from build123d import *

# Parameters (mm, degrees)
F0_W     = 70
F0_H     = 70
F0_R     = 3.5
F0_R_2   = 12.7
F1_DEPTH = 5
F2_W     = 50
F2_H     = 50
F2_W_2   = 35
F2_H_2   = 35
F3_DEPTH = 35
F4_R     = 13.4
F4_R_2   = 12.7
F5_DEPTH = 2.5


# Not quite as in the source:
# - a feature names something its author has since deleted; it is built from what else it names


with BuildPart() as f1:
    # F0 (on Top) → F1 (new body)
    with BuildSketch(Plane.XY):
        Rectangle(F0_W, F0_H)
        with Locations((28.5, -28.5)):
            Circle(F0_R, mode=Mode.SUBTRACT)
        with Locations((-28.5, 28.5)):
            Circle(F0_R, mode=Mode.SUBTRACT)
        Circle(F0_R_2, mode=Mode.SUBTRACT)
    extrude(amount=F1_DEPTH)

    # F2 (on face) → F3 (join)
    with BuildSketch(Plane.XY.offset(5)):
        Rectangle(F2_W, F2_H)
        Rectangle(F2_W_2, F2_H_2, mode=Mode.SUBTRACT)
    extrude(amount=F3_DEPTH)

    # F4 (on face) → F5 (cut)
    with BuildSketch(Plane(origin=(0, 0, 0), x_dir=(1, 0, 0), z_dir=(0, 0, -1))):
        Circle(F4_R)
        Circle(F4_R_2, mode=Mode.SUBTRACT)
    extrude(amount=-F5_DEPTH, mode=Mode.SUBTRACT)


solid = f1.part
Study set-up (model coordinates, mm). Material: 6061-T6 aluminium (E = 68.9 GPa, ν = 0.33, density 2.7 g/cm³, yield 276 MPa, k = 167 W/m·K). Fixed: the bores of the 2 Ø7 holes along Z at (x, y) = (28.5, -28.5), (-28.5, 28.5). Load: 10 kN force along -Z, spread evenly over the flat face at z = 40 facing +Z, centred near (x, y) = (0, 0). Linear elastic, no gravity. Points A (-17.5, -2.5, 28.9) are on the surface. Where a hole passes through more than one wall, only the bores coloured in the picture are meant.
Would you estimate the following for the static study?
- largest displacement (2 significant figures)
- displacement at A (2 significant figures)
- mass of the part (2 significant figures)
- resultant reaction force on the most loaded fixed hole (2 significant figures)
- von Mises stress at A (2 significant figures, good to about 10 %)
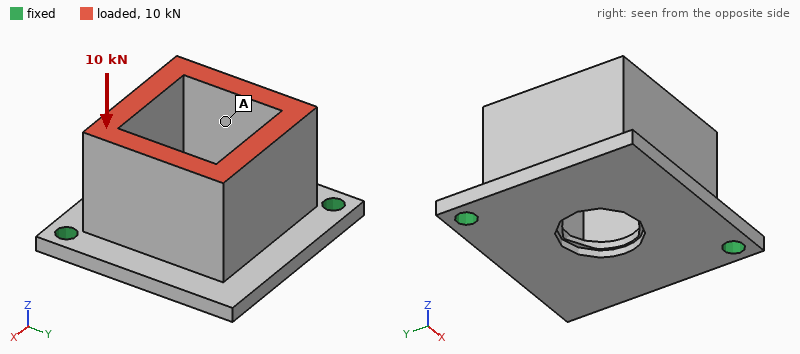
0.15 mm
0.094 mm
180 g
5.6 kN
22 MPa
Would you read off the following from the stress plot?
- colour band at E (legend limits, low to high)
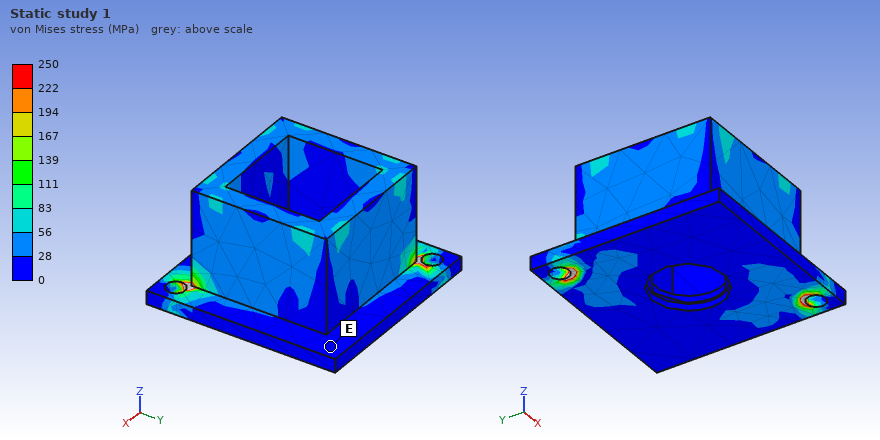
0 to 28 MPa
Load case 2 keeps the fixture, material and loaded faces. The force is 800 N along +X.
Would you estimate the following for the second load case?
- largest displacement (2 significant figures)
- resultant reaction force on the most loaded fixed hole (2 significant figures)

0.17 mm
500 N
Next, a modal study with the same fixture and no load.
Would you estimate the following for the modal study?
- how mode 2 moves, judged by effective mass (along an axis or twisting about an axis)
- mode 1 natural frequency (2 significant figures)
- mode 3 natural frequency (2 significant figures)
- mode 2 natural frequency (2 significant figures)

along Z
1200 Hz
7400 Hz
3800 Hz
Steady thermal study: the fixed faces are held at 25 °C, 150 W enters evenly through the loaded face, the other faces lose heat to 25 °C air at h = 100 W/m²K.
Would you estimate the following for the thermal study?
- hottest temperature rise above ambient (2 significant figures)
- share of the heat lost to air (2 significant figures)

49 K
44 %
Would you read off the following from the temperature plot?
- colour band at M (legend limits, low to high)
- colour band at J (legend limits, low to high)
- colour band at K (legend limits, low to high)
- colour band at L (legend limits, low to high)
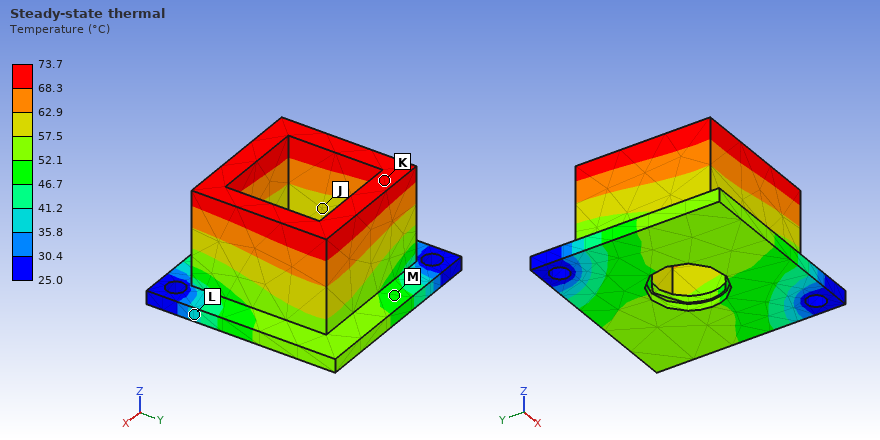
46.7 to 52.1 °C
57.5 to 62.9 °C
68.3 to 73.7 °C
35.8 to 41.2 °C
